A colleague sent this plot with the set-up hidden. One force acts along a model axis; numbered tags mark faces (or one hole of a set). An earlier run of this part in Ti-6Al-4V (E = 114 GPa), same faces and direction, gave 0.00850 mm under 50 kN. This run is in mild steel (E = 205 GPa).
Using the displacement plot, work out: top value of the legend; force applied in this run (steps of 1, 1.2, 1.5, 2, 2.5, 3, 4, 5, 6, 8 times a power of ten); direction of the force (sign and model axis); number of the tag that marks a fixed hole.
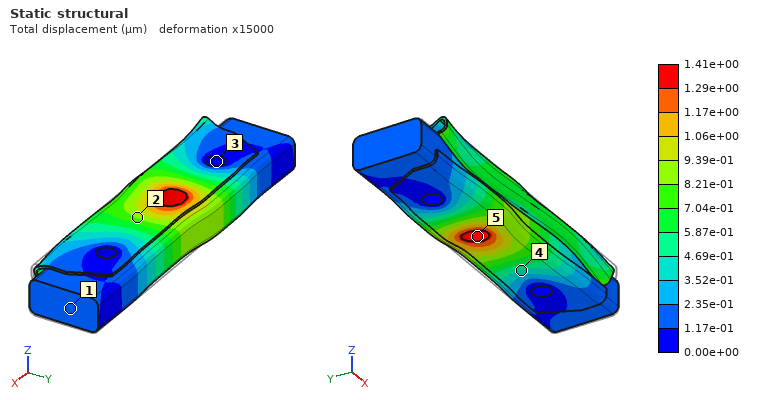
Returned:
1.41e+00 µm
15 kN
-X
3
